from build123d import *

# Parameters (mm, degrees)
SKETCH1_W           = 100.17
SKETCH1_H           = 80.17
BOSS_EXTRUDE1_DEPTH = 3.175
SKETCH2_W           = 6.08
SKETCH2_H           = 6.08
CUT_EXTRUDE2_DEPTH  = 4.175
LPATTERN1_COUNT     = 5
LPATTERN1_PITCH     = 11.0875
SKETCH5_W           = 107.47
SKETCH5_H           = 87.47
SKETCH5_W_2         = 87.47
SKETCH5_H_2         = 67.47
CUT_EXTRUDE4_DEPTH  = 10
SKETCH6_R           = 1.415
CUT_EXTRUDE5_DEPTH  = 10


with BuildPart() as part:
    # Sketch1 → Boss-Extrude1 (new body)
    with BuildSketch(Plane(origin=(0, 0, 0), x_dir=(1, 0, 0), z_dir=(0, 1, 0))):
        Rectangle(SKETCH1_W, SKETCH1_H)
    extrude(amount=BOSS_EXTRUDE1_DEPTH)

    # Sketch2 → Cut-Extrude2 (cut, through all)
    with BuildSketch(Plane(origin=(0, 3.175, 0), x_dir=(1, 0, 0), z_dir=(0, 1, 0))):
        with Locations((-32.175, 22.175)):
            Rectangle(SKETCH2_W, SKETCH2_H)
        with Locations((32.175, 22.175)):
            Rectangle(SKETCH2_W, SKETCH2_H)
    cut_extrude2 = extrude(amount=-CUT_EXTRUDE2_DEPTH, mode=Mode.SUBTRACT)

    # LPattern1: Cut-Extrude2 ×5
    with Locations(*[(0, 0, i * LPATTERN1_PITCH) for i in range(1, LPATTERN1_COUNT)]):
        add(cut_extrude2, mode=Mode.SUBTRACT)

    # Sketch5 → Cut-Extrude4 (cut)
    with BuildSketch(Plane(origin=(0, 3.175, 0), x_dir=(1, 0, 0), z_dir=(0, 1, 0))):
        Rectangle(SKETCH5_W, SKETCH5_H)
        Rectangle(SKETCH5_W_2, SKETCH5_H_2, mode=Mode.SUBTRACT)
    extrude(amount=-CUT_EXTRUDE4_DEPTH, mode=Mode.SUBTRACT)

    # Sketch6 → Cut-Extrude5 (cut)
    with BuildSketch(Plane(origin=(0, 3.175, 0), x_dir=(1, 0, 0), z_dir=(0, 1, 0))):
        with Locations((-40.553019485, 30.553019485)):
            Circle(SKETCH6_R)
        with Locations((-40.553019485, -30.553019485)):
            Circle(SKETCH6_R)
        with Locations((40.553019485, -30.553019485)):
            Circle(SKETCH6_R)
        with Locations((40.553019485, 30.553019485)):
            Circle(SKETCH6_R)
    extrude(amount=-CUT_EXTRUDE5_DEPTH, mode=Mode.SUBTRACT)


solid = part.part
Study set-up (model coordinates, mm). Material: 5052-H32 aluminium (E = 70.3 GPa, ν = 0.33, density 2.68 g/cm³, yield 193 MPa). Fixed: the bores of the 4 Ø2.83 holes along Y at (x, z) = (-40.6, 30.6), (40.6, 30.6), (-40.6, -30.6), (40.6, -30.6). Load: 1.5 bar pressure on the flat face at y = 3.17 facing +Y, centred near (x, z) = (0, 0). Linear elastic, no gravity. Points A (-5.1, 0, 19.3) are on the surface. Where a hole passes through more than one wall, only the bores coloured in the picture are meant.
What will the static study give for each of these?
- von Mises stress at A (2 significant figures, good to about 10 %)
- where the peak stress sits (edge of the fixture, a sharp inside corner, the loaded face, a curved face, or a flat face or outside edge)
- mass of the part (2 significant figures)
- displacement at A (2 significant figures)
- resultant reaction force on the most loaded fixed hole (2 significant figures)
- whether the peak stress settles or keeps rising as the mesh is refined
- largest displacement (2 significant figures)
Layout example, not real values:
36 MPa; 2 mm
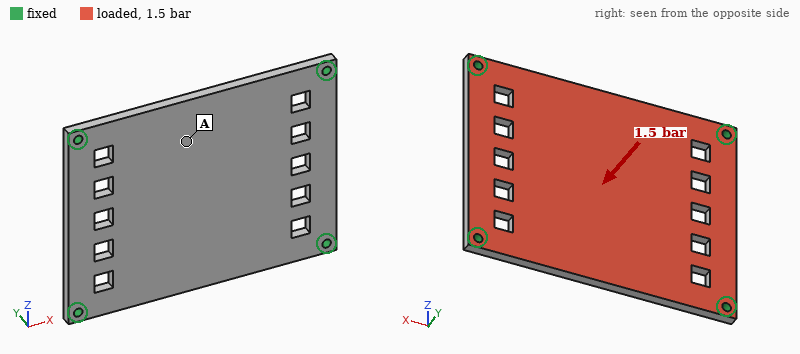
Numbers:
31 MPa; edge of the fixture; 47 g; 0.17 mm; 210 N; keeps rising; 0.19 mm
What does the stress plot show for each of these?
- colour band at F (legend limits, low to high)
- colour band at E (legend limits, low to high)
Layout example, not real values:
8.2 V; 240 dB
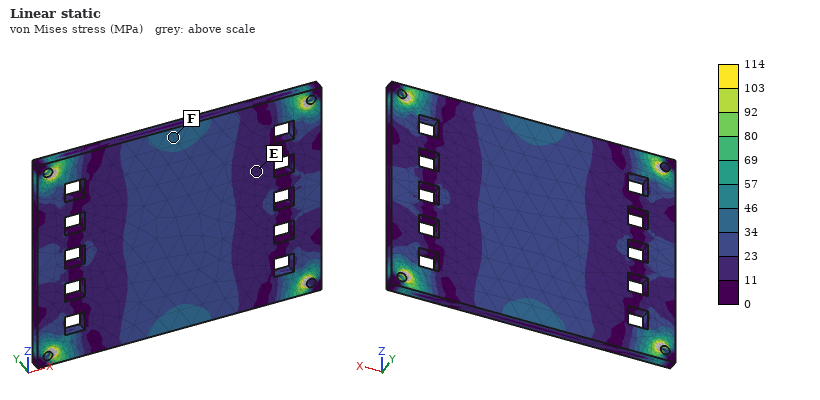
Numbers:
34 to 46 MPa; 11 to 23 MPa
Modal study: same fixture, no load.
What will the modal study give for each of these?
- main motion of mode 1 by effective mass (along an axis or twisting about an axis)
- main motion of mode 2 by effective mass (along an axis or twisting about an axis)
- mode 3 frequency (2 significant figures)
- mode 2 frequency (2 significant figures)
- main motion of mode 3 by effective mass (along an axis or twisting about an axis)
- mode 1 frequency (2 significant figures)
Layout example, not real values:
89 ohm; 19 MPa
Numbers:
along Y; twisting about X; 4000 Hz; 2900 Hz; twisting about Z; 1800 Hz
